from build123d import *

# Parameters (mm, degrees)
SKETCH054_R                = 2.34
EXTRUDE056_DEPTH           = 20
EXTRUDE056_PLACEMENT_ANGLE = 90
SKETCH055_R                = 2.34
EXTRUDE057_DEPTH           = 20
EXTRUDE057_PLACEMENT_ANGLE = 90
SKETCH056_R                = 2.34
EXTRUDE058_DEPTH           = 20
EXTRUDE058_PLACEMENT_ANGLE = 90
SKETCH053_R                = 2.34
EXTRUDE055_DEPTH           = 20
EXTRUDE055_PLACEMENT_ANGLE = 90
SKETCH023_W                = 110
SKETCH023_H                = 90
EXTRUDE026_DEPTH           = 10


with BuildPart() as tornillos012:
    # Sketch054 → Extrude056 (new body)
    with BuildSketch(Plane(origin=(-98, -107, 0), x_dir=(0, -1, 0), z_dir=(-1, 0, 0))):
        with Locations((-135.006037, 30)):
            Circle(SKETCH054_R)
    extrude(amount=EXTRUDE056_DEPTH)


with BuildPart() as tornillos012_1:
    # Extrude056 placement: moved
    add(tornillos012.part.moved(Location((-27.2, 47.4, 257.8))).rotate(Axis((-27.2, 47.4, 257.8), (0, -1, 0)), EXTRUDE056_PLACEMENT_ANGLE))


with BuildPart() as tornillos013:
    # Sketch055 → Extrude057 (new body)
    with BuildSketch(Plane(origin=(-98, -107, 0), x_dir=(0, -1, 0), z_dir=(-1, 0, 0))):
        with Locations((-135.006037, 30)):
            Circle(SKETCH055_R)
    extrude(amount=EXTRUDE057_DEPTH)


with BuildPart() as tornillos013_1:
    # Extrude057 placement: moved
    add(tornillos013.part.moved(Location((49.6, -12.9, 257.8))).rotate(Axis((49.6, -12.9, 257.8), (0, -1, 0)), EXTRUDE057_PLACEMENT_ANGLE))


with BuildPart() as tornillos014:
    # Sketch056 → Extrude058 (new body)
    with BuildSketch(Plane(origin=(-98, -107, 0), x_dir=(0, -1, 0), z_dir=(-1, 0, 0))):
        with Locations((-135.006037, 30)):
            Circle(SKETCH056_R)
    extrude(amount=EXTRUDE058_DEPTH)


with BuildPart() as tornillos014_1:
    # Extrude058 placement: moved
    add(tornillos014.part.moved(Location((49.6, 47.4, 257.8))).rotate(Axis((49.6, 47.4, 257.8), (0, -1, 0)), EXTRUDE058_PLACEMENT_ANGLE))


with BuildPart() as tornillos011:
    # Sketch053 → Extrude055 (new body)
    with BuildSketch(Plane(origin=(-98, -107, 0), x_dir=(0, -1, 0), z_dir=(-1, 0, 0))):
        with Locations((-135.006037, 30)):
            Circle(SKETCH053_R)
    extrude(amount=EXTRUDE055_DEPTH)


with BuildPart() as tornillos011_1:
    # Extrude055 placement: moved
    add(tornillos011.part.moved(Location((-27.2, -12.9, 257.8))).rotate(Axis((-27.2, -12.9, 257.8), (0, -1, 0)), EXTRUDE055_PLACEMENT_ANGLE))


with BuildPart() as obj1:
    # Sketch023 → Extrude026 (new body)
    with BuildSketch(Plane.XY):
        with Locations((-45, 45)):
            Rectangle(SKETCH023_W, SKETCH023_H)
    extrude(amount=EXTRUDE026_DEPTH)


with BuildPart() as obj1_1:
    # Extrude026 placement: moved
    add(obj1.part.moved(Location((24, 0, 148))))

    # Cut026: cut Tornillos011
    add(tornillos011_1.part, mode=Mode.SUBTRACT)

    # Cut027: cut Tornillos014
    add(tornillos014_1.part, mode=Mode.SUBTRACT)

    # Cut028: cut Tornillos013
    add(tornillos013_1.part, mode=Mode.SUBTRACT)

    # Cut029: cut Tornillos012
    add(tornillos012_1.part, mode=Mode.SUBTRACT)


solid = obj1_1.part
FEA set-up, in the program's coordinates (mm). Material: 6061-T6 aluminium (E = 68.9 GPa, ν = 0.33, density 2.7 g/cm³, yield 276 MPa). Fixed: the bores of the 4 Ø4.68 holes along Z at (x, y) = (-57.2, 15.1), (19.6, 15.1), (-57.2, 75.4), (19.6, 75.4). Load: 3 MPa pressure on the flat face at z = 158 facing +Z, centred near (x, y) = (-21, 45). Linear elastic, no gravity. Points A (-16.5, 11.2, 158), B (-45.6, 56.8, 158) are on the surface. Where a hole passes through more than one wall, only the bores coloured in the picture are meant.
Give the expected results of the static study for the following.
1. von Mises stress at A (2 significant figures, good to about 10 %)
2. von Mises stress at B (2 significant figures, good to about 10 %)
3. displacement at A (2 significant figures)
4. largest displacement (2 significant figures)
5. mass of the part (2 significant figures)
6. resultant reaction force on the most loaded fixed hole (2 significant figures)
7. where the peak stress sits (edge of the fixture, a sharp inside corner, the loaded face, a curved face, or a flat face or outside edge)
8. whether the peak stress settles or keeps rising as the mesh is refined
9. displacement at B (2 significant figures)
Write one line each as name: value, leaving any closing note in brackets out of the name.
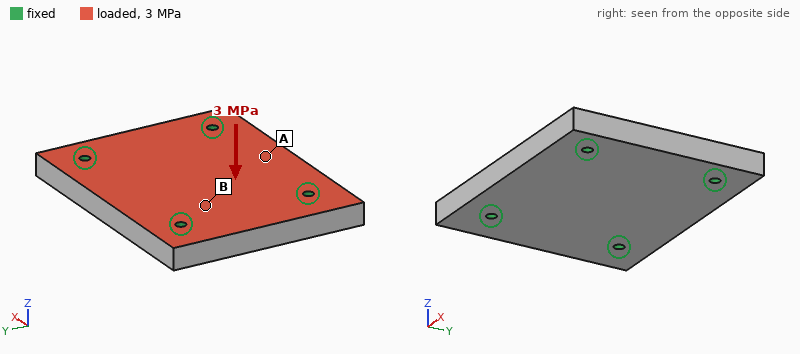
von Mises stress at A: 52 MPa
von Mises stress at B: 24 MPa
displacement at A: 78 µm
largest displacement: 98 µm
mass of the part: 270 g
resultant reaction force on the most loaded fixed hole: 7.8 kN
where the peak stress sits: edge of the fixture
whether the peak stress settles or keeps rising as the mesh is refined: keeps rising
displacement at B: 57 µm
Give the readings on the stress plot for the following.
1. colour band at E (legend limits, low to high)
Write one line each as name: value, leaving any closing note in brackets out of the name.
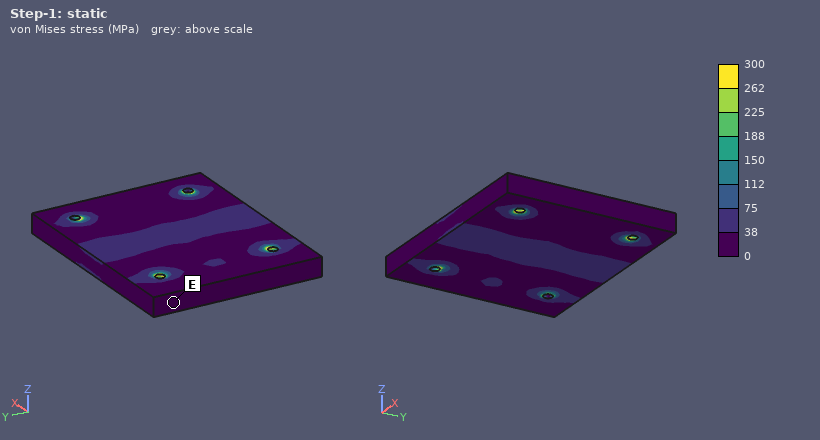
colour band at E: 0 to 38 MPa
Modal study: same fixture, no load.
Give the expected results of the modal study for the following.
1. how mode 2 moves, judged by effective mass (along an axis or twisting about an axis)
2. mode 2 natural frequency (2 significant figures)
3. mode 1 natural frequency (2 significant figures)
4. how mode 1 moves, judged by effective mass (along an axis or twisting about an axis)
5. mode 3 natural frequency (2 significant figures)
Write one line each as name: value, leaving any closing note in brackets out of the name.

how mode 2 moves, judged by effective mass: twisting about X
mode 2 natural frequency: 8100 Hz
mode 1 natural frequency: 6200 Hz
how mode 1 moves, judged by effective mass: along Z
mode 3 natural frequency: 9400 Hz
